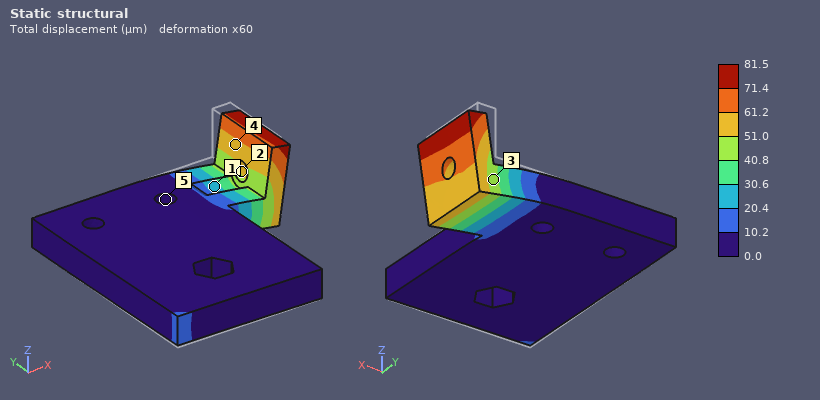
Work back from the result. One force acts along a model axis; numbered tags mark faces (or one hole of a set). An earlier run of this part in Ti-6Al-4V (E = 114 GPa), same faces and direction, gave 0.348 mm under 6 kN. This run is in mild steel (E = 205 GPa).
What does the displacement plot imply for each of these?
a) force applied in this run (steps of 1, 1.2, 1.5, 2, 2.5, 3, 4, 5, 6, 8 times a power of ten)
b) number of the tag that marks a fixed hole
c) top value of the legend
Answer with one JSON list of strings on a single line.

["2.5 kN", "5", "81.5 µm"]
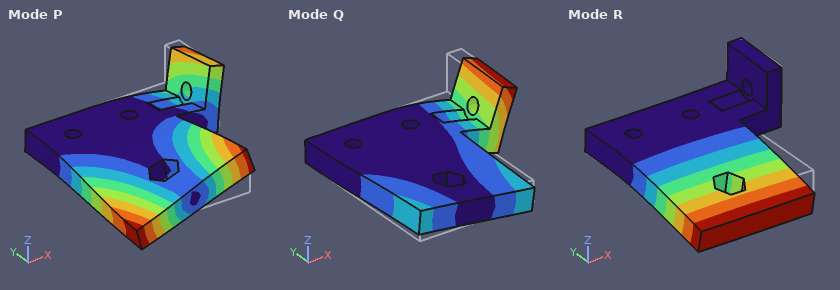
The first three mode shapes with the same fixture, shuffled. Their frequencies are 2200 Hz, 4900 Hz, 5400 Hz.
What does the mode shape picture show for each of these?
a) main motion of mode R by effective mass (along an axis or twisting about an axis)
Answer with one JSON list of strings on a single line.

["along Z"]
